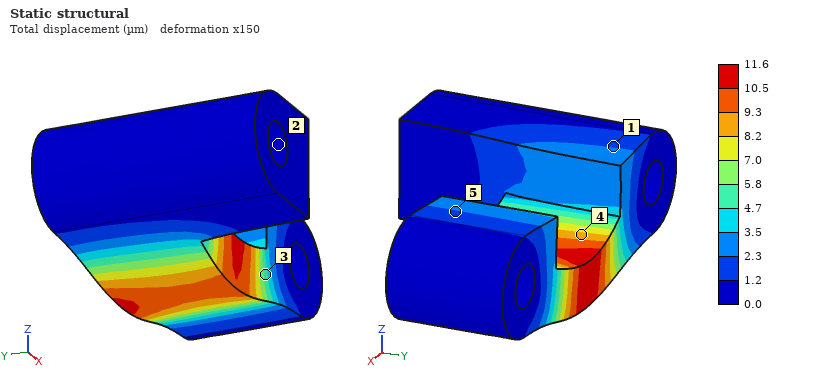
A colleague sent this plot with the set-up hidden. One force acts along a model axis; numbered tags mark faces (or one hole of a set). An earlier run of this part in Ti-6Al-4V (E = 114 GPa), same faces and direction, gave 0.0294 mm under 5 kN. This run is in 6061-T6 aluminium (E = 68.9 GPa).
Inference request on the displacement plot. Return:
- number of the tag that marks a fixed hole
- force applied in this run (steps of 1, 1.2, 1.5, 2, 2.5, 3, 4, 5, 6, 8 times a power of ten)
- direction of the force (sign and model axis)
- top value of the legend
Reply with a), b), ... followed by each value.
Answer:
a) 2
b) 1.2 kN
c) -Z
d) 11.6 µm
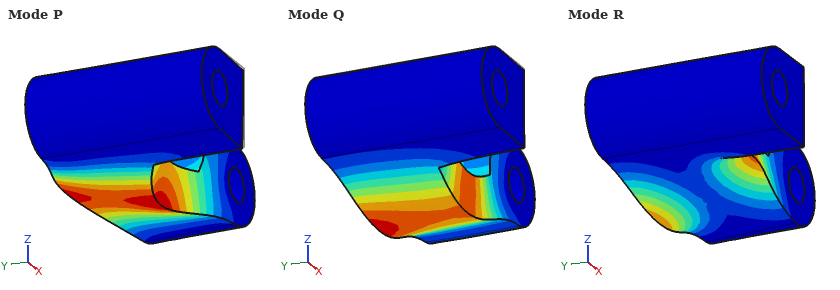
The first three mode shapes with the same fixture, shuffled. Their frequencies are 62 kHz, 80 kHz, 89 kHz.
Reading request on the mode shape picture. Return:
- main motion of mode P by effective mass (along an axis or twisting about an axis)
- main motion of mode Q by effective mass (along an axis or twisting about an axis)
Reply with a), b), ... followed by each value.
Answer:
a) along Y
b) along Z
